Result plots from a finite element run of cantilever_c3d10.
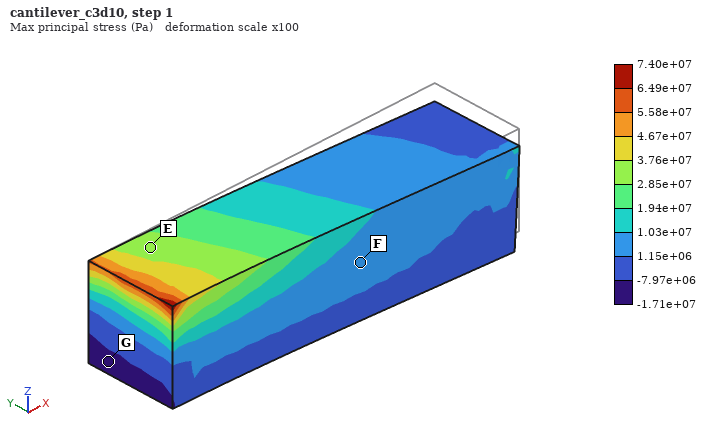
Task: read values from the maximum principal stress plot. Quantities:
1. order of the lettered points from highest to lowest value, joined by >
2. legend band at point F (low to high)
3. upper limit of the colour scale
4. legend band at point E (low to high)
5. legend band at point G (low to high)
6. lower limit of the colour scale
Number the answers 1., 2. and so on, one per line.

1. E > F > G
2. 1.15e+06 to 1.03e+07 Pa
3. 7.40e+07 Pa
4. 2.85e+07 to 3.76e+07 Pa
5. -1.71e+07 to -7.97e+06 Pa
6. -1.71e+07 Pa
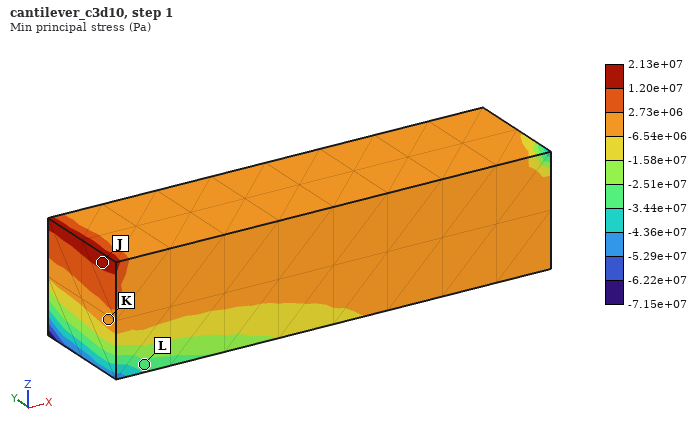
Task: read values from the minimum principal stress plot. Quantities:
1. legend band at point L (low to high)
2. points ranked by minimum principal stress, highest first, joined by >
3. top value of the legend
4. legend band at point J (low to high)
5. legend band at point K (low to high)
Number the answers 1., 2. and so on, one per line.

1. -3.44e+07 to -2.51e+07 Pa
2. J > K > L
3. 2.13e+07 Pa
4. 1.20e+07 to 2.13e+07 Pa
5. -6.54e+06 to 2.73e+06 Pa
